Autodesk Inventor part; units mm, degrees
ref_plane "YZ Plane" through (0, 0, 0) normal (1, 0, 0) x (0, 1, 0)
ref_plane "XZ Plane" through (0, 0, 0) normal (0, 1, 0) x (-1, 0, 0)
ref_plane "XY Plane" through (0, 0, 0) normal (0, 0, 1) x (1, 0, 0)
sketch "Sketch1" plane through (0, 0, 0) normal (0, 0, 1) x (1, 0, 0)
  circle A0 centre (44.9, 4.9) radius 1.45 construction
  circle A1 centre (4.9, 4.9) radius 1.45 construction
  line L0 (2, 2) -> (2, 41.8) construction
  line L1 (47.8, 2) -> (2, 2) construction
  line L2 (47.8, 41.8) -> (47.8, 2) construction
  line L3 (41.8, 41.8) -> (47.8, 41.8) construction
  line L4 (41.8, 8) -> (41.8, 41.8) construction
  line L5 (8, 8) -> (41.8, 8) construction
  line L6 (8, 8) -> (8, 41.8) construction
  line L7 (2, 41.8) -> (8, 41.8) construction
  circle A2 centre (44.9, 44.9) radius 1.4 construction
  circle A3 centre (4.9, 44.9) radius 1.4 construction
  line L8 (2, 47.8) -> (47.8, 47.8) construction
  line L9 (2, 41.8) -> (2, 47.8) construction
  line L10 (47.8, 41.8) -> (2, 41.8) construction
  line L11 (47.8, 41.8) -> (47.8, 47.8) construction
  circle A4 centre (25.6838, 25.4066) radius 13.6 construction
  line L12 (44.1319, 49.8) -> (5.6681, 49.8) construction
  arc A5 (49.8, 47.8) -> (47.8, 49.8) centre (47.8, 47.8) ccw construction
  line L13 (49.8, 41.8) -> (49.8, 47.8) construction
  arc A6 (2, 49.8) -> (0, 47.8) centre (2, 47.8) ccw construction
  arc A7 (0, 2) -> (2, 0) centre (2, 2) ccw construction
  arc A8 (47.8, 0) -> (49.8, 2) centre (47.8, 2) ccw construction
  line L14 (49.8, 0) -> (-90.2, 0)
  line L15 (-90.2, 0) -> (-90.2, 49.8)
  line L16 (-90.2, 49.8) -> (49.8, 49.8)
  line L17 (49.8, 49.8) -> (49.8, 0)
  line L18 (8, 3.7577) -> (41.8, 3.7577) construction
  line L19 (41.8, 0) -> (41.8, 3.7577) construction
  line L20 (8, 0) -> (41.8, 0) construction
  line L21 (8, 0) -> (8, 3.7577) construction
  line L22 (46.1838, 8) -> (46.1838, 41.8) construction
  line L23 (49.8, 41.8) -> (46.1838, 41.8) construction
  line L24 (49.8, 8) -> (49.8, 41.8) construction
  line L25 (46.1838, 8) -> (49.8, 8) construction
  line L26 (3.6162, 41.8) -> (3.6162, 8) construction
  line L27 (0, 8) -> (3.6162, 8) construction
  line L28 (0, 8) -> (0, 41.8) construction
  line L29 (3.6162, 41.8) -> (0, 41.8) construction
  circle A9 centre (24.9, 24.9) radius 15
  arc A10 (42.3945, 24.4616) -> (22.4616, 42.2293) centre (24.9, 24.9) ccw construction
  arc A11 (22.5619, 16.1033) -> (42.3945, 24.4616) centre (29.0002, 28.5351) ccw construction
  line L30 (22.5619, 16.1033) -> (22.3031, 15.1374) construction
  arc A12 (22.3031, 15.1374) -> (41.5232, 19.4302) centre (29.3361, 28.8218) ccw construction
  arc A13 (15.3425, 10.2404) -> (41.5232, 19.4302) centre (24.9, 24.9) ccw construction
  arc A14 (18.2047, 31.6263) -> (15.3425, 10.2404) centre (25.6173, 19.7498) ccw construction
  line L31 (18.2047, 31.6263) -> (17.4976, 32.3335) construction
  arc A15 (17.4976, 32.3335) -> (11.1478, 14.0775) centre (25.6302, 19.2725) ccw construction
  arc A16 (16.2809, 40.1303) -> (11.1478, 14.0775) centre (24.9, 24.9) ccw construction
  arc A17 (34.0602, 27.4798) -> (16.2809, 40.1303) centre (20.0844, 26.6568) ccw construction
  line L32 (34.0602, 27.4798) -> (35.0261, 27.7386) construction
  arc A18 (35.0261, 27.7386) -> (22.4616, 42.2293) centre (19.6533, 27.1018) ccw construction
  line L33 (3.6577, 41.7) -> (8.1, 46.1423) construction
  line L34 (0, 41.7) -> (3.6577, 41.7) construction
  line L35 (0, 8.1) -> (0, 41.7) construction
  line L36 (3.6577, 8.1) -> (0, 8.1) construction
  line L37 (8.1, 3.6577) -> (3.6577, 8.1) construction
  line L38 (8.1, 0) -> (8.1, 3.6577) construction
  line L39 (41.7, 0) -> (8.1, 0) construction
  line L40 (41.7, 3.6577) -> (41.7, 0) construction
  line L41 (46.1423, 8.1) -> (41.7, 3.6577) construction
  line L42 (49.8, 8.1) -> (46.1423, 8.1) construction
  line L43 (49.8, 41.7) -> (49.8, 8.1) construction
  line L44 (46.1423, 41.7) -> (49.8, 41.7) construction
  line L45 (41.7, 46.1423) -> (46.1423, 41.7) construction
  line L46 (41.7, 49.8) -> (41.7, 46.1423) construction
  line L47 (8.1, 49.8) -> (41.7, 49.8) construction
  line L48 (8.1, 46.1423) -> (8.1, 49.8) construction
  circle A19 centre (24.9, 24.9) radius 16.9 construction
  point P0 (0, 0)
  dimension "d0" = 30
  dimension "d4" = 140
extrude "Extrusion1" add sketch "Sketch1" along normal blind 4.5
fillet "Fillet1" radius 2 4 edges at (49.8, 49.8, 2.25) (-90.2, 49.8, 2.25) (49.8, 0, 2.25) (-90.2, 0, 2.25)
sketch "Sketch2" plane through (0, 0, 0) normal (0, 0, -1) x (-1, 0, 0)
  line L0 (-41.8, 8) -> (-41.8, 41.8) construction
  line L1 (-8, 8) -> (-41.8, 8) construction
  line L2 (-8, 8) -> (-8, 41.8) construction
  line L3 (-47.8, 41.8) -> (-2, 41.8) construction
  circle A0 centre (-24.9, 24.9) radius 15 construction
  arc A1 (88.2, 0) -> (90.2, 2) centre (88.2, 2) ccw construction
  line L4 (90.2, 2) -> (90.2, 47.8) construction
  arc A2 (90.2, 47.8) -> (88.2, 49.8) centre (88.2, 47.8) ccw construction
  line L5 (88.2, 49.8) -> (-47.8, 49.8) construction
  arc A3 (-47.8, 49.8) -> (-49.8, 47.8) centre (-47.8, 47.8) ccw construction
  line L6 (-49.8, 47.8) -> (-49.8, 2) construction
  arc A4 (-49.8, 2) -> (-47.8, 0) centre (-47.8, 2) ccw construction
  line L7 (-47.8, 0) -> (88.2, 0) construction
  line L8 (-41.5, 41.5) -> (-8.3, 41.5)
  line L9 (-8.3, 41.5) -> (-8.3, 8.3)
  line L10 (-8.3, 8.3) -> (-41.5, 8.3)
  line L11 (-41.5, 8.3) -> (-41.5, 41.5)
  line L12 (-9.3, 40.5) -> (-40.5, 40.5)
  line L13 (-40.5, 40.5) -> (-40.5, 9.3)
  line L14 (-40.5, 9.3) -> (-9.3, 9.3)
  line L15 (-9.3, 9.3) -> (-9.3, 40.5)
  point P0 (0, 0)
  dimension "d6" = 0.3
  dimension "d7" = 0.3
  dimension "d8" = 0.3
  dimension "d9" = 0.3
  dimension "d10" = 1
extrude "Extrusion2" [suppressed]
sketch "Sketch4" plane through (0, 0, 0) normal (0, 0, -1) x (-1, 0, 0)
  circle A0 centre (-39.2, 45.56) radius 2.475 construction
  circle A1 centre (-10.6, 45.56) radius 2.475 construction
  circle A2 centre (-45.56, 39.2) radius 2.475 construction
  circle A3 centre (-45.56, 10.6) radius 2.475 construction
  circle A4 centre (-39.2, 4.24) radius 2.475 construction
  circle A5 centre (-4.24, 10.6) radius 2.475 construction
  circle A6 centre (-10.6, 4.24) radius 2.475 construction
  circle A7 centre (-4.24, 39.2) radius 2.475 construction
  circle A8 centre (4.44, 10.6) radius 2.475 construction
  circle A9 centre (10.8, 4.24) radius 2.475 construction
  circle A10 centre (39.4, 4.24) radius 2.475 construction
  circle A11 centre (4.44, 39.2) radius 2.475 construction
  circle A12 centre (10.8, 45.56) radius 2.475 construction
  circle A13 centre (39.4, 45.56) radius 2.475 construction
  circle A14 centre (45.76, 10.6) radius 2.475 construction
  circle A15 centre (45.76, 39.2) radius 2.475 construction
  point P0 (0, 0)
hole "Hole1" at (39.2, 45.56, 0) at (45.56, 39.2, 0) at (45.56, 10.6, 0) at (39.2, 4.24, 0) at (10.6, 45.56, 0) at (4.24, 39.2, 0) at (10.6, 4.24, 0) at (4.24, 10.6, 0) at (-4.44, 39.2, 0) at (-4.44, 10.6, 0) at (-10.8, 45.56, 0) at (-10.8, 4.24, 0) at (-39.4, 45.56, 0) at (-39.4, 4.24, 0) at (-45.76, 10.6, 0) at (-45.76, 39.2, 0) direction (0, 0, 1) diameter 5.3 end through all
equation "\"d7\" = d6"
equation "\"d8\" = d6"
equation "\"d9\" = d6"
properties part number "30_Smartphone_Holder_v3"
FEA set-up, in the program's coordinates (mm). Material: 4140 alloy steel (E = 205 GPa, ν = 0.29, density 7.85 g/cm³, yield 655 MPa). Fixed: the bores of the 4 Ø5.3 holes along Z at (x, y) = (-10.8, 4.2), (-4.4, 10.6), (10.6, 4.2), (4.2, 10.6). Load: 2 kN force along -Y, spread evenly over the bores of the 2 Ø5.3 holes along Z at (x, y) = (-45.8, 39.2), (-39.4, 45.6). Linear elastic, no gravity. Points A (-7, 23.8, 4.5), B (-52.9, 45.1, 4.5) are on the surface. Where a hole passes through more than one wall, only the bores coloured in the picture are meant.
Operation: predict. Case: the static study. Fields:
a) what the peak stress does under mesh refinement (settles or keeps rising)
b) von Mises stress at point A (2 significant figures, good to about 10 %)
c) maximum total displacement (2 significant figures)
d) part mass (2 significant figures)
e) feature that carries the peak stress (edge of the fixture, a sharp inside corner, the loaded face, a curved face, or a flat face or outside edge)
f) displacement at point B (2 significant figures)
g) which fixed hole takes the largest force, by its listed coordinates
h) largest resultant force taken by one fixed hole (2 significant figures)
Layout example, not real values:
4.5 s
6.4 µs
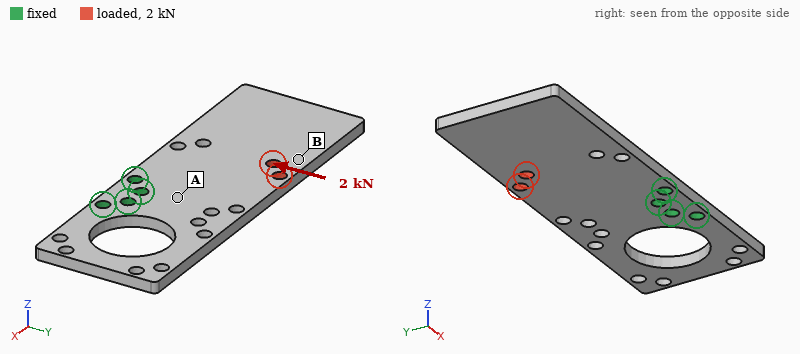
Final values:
keeps rising
29 MPa
49 µm
210 g
edge of the fixture
32 µm
(-10.8, 4.2)
3.8 kN
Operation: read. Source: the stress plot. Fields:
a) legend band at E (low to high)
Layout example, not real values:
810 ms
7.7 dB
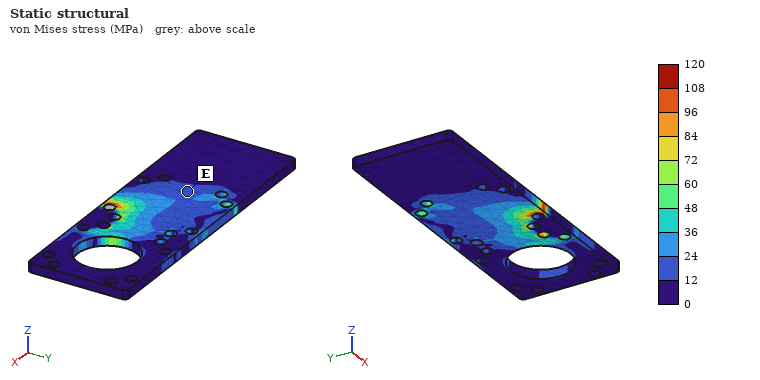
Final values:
12 to 24 MPa
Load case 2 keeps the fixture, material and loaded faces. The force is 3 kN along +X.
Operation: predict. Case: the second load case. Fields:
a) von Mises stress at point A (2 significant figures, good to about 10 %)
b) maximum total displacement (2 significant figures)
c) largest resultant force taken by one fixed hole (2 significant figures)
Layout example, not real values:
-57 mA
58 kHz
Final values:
52 MPa
69 µm
3.4 kN
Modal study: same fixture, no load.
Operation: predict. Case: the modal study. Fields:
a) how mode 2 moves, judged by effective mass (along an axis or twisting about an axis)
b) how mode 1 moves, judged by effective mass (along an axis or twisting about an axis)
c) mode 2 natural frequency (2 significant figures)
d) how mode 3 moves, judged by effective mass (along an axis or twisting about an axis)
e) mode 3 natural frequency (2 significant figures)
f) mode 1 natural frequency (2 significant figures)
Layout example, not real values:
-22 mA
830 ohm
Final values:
along Z
along Z
1300 Hz
twisting about X
1500 Hz
480 Hz
